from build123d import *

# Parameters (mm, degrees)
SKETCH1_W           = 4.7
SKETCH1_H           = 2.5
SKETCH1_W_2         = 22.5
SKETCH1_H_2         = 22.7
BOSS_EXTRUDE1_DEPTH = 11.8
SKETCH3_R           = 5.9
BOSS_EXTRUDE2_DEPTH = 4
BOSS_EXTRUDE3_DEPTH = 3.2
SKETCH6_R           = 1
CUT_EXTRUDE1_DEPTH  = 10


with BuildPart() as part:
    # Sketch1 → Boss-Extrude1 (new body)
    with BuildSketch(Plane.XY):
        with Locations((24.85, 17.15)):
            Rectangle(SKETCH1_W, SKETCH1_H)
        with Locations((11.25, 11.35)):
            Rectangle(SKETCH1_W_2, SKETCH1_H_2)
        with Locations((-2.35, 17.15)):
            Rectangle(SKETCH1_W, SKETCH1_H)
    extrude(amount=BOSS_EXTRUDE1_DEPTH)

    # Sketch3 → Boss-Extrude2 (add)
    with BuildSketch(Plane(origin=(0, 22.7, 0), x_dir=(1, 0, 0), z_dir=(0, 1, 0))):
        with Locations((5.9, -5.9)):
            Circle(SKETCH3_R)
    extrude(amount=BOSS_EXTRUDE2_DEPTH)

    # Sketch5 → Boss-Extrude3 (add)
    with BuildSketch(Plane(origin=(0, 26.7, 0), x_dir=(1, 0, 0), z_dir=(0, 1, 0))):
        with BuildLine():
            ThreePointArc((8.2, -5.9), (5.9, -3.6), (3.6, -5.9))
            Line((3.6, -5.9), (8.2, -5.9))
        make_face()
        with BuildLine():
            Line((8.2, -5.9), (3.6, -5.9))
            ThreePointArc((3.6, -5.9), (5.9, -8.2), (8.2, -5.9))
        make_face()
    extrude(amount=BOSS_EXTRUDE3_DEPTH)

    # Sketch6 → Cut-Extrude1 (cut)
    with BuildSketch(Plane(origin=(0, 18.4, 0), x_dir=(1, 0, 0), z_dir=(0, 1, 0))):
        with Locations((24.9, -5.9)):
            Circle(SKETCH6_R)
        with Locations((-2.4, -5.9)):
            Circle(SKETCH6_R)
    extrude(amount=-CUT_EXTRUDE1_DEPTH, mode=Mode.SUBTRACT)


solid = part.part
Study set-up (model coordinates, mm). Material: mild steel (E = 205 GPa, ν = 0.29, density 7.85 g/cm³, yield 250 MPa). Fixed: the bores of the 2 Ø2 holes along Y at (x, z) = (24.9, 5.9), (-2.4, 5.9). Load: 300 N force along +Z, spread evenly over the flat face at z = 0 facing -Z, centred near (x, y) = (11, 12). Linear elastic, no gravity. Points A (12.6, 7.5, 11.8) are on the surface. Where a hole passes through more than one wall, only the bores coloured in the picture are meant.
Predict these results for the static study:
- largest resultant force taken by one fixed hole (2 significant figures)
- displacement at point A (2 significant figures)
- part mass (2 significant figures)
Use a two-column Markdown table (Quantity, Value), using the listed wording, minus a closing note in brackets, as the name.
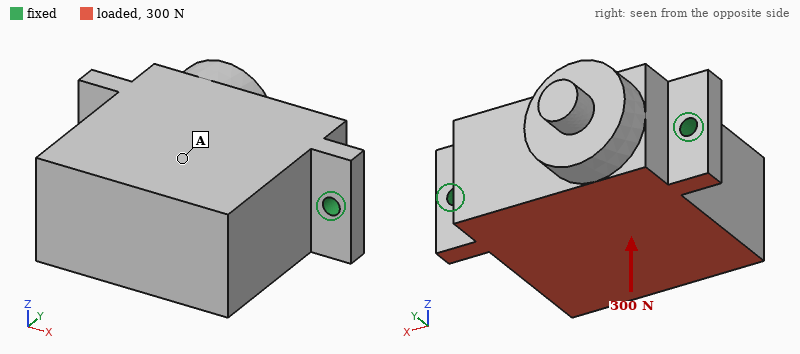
| Quantity | Value |
|---|---|
| largest resultant force taken by one fixed hole | 150 N |
| displacement at point A | 7.1 µm |
| part mass | 53 g |
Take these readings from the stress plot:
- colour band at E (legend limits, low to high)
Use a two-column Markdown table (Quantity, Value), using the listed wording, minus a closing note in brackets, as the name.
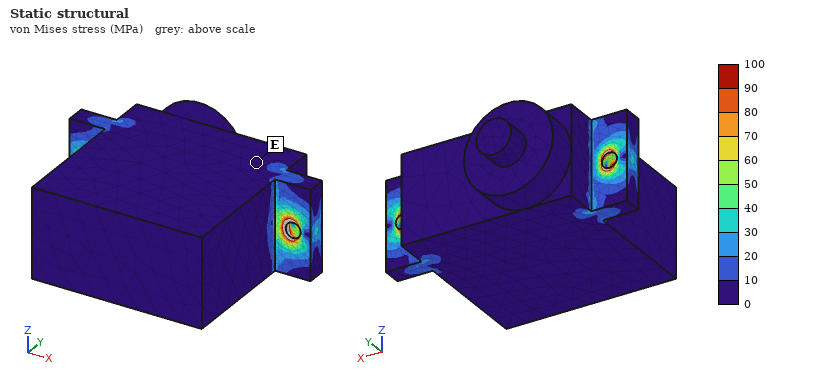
| Quantity | Value |
|---|---|
| colour band at E | 0 to 10 MPa |
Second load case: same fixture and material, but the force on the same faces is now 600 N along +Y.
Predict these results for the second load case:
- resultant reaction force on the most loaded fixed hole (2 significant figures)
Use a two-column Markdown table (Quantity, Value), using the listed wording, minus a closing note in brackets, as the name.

| Quantity | Value |
|---|---|
| resultant reaction force on the most loaded fixed hole | 300 N |
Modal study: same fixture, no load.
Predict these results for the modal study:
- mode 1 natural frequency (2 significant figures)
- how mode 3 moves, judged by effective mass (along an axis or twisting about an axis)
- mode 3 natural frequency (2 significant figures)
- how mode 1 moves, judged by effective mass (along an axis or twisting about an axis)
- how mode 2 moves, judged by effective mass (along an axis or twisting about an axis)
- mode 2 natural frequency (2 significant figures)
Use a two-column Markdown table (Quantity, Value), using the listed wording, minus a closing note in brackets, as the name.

| Quantity | Value |
|---|---|
| mode 1 natural frequency | 4000 Hz |
| how mode 3 moves, judged by effective mass | along X |
| mode 3 natural frequency | 17 kHz |
| how mode 1 moves, judged by effective mass | along Z |
| how mode 2 moves, judged by effective mass | along Y |
| mode 2 natural frequency | 16 kHz |
